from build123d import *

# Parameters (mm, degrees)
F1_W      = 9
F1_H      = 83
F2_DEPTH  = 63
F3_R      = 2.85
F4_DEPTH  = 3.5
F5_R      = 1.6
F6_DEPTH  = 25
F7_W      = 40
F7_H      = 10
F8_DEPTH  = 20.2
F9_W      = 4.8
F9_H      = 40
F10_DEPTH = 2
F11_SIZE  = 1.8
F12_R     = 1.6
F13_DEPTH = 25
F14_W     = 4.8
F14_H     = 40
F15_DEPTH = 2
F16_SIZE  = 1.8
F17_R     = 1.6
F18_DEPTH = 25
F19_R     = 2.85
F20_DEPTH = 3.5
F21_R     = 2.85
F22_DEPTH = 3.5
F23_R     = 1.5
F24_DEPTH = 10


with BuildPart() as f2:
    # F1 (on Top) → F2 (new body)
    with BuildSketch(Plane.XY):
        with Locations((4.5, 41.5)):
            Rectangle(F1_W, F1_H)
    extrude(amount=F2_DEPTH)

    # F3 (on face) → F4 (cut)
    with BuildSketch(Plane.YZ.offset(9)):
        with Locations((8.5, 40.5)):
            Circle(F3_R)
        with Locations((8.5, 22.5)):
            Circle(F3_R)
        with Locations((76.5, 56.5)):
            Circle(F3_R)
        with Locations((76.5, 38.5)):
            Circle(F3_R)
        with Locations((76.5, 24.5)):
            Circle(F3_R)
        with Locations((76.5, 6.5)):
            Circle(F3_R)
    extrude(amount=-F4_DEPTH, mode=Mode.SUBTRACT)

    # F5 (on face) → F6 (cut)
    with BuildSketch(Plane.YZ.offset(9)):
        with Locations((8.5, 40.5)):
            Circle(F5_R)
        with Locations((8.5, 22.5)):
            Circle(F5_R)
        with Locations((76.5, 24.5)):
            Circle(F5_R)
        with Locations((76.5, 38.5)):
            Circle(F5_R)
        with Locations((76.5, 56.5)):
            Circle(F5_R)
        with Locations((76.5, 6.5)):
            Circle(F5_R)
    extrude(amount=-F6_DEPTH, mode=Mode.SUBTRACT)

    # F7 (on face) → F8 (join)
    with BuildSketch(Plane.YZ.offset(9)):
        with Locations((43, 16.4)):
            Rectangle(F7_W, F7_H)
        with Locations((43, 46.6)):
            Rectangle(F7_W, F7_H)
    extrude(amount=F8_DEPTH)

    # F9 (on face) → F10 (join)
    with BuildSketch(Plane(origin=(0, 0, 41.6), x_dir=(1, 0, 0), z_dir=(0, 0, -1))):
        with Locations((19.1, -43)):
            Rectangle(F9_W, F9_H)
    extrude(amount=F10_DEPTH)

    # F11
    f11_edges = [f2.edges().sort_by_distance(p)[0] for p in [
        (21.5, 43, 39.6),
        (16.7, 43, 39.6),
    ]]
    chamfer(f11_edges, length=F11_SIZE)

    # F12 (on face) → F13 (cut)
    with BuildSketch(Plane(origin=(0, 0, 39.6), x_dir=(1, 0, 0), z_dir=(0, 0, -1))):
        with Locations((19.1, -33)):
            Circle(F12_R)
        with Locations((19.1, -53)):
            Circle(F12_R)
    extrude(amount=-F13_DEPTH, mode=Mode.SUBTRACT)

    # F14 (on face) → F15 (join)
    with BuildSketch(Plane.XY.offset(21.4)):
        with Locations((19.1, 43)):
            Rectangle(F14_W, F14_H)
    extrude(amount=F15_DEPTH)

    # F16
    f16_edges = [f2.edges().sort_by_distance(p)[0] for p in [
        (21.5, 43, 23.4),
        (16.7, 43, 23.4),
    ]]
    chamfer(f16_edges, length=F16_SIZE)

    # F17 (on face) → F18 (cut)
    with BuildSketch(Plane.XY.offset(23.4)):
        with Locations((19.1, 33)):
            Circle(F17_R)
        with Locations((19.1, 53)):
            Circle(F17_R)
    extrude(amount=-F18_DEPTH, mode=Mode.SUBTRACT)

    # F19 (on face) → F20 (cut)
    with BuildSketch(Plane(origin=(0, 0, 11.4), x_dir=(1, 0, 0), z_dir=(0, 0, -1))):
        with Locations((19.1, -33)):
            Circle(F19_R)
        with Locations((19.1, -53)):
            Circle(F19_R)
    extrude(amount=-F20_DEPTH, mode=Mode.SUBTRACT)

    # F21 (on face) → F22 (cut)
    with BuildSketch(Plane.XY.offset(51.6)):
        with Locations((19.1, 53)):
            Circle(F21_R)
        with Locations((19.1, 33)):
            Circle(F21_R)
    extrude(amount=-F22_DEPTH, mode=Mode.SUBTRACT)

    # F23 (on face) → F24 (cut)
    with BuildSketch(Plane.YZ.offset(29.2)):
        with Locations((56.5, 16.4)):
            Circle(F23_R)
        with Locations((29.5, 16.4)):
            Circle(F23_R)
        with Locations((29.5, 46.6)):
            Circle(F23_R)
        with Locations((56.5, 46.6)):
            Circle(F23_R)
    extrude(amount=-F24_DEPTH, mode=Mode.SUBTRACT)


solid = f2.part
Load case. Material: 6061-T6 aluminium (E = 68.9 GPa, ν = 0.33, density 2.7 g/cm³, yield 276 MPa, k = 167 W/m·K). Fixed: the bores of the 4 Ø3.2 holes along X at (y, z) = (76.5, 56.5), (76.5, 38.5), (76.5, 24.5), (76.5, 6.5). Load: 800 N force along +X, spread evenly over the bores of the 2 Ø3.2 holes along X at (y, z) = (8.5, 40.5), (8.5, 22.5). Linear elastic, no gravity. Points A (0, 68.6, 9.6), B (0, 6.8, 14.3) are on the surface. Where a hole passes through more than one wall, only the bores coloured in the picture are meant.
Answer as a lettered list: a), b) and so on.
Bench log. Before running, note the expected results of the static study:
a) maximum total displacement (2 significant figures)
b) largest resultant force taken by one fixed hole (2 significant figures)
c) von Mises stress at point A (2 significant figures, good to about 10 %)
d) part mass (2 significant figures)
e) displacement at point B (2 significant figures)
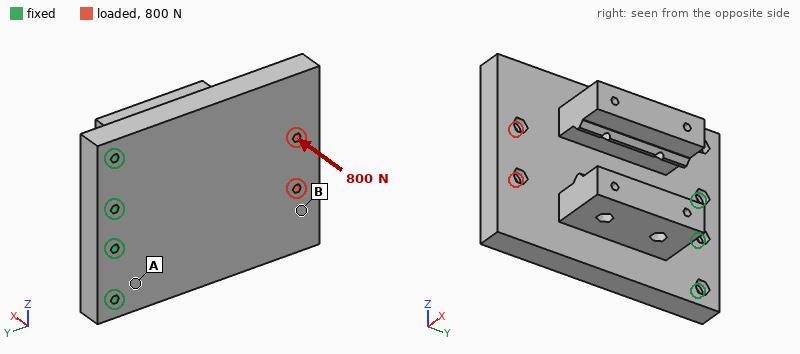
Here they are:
a) 0.42 mm
b) 380 N
c) 52 MPa
d) 170 g
e) 0.37 mm
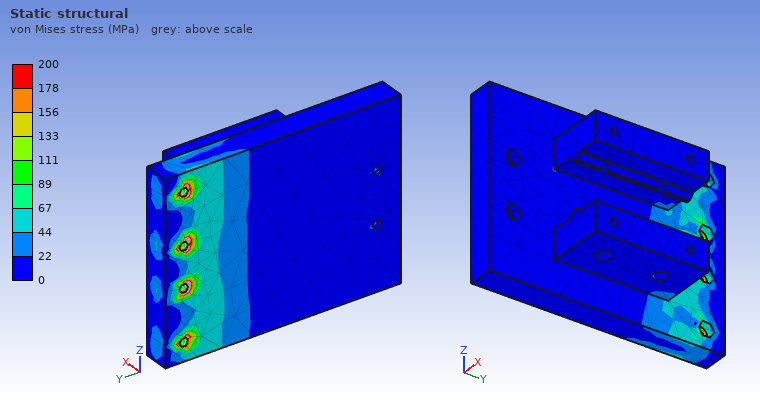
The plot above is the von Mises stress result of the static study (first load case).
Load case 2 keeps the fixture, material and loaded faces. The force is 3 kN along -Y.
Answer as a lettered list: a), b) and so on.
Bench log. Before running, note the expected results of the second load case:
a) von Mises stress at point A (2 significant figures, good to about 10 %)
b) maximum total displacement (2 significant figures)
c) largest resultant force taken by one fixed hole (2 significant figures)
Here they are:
a) 12 MPa
b) 43 µm
c) 790 N
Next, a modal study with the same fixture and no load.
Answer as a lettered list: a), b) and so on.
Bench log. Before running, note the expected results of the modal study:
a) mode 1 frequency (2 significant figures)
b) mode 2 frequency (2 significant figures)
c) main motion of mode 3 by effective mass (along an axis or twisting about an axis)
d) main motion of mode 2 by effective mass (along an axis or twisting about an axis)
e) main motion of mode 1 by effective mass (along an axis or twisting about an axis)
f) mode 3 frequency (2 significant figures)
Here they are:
a) 990 Hz
b) 3000 Hz
c) along Z
d) twisting about Y
e) along X
f) 5100 Hz
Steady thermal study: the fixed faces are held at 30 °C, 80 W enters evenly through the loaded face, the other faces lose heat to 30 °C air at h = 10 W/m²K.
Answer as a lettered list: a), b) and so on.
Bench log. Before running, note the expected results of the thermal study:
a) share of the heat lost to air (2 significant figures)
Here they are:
a) 6.1 %
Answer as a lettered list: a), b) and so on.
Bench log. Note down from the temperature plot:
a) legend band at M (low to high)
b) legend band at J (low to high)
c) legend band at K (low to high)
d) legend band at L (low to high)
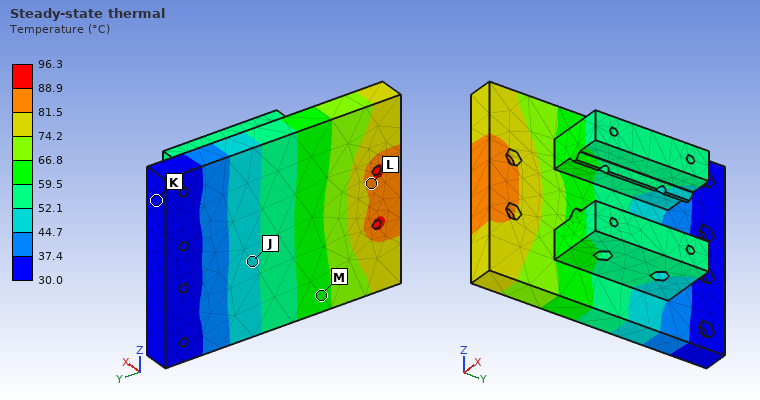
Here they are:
a) 59.5 to 66.8 °C
b) 44.7 to 52.1 °C
c) 30.0 to 37.4 °C
d) 81.5 to 88.9 °C
